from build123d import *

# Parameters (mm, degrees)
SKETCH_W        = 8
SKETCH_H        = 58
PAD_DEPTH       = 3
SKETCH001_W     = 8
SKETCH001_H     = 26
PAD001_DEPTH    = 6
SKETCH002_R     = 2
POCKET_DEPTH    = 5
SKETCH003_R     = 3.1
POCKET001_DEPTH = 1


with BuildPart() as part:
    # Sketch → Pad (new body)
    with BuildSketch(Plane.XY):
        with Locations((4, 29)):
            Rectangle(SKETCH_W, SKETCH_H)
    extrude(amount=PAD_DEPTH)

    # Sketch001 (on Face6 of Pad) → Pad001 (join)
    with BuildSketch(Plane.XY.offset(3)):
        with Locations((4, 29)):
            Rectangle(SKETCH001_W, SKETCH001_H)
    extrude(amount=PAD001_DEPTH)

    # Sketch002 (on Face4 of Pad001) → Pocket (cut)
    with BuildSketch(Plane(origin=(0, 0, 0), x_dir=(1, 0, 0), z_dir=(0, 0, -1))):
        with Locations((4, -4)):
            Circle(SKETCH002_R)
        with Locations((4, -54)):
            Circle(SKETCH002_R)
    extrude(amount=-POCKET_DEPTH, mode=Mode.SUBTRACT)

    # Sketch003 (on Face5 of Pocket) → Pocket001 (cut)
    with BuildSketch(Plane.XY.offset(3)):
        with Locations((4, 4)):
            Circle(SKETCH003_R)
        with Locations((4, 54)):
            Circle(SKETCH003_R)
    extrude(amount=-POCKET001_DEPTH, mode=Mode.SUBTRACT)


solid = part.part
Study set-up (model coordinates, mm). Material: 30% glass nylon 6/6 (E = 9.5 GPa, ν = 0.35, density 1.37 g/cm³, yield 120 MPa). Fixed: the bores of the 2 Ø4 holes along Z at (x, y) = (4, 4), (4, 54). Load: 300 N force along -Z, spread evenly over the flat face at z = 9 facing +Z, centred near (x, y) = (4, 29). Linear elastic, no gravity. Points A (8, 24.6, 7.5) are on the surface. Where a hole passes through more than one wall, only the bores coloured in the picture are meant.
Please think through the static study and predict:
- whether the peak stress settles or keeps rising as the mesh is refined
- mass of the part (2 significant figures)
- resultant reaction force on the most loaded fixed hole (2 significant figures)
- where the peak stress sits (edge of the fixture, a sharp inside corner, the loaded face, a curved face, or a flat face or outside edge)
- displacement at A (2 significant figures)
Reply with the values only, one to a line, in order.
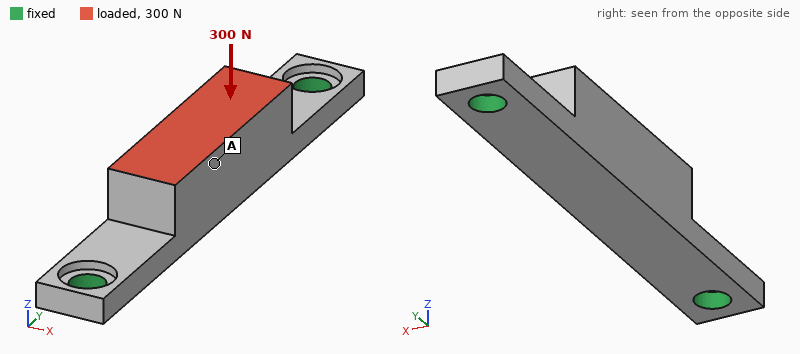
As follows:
keeps rising
3.5 g
260 N
edge of the fixture
0.22 mm
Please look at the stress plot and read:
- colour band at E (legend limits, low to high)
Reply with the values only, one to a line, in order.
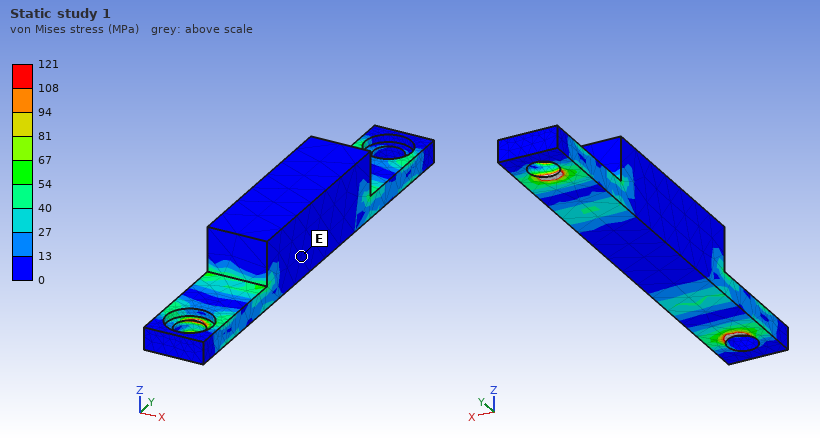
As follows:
0 to 13 MPa
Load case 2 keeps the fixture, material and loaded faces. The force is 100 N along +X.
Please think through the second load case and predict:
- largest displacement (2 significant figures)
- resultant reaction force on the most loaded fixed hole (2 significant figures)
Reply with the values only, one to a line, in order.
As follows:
0.24 mm
50 N
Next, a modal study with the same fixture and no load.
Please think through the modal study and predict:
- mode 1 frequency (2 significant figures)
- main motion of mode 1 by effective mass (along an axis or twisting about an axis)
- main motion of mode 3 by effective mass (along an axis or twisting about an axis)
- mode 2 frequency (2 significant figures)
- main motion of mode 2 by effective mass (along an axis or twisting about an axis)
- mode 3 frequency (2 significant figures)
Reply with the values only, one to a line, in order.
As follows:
3300 Hz
along X
along X
3600 Hz
along Z
7400 Hz
